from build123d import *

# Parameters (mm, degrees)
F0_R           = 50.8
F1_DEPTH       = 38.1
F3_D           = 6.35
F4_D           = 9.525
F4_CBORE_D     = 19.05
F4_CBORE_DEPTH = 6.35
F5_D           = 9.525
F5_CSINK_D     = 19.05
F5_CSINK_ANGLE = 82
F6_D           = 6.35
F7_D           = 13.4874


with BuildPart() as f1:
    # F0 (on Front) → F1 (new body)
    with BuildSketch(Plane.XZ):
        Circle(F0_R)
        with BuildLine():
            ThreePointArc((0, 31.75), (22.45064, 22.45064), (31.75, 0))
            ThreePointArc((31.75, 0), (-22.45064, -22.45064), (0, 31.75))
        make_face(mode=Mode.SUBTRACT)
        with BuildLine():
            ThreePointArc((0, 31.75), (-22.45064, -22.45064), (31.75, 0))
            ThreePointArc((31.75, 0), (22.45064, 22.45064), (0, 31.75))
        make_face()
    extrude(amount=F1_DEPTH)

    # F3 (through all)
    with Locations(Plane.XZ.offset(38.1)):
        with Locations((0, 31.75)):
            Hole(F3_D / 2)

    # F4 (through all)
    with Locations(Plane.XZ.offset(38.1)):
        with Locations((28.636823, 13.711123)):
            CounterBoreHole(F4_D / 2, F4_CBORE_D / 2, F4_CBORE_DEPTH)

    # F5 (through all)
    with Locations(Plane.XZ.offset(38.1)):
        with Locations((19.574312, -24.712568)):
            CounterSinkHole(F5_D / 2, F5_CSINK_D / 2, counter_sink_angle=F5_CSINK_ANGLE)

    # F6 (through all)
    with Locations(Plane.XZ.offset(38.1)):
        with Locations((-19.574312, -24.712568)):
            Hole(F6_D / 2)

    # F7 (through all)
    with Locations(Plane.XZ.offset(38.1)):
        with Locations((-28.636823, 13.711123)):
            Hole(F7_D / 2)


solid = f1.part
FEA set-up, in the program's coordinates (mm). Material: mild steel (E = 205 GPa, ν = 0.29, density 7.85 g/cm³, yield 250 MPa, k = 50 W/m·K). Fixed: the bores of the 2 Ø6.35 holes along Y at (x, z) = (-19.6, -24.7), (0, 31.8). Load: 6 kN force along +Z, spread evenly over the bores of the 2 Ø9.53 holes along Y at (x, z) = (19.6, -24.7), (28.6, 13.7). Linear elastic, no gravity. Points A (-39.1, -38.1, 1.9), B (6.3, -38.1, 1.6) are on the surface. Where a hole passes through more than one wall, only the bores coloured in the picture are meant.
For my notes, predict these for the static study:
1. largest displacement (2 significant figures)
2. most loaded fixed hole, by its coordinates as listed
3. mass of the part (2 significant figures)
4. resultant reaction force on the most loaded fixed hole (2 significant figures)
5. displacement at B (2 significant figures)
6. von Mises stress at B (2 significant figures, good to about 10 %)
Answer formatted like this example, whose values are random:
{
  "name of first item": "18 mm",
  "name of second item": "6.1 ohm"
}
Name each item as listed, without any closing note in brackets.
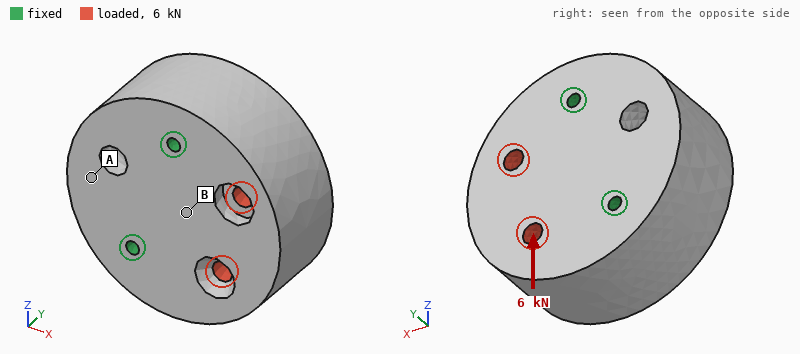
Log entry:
{
  "largest displacement": "1.6 µm",
  "most loaded fixed hole, by its coordinates as listed": "(0, 31.8)",
  "mass of the part": "2.3 kg",
  "resultant reaction force on the most loaded fixed hole": "5.2 kN",
  "displacement at B": "0.50 µm",
  "von Mises stress at B": "3.0 MPa"
}
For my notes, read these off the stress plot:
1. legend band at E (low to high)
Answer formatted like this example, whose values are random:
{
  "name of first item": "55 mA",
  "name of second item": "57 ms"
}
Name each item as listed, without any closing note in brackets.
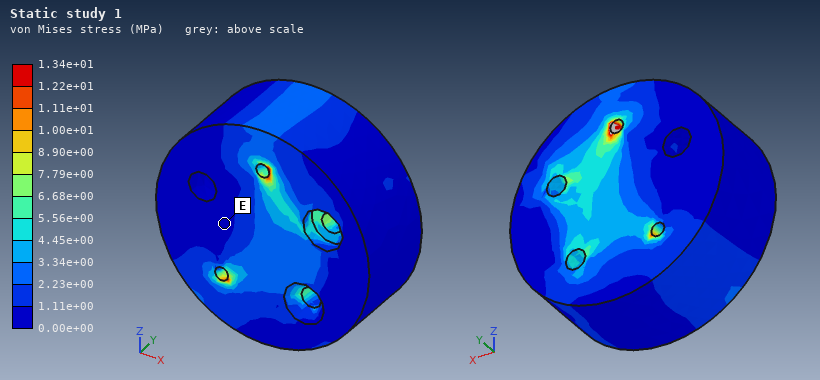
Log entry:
{
  "legend band at E": "0.00e+00 to 1.11e+00 MPa"
}
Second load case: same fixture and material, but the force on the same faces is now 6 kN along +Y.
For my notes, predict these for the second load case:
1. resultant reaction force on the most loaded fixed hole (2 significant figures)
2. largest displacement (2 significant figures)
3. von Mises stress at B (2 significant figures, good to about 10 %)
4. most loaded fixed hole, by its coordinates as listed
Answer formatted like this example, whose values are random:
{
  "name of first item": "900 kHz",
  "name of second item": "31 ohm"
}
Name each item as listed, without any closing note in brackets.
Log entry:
{
  "resultant reaction force on the most loaded fixed hole": "3.2 kN",
  "largest displacement": "5.3 µm",
  "von Mises stress at B": "3.7 MPa",
  "most loaded fixed hole, by its coordinates as listed": "(0, 31.8)"
}
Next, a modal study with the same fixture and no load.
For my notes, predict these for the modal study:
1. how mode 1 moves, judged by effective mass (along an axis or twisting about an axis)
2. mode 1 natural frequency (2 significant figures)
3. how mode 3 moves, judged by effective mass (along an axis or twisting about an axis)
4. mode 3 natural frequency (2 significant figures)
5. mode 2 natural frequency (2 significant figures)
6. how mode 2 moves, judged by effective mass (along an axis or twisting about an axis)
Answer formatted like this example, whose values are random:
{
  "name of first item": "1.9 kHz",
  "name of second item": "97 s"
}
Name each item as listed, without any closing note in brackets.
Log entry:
{
  "how mode 1 moves, judged by effective mass": "along Y",
  "mode 1 natural frequency": "6300 Hz",
  "how mode 3 moves, judged by effective mass": "along Y",
  "mode 3 natural frequency": "12 kHz",
  "mode 2 natural frequency": "10 kHz",
  "how mode 2 moves, judged by effective mass": "along Z"
}
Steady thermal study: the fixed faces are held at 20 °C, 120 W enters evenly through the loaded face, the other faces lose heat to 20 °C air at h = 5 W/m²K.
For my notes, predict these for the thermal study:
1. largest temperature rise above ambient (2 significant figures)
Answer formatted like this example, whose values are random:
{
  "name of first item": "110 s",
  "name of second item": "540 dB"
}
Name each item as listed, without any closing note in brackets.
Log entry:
{
  "largest temperature rise above ambient": "36 K"
}
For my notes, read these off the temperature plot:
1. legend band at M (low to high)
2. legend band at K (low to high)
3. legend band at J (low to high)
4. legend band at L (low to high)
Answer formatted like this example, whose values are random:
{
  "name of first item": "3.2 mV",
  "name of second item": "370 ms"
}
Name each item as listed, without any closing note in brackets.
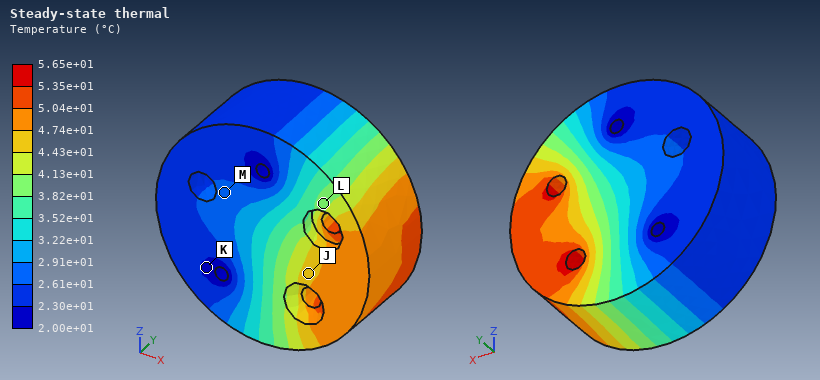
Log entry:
{
  "legend band at M": "2.61e+01 to 2.91e+01 °C",
  "legend band at K": "2.00e+01 to 2.30e+01 °C",
  "legend band at J": "4.43e+01 to 4.74e+01 °C",
  "legend band at L": "3.82e+01 to 4.13e+01 °C"
}
